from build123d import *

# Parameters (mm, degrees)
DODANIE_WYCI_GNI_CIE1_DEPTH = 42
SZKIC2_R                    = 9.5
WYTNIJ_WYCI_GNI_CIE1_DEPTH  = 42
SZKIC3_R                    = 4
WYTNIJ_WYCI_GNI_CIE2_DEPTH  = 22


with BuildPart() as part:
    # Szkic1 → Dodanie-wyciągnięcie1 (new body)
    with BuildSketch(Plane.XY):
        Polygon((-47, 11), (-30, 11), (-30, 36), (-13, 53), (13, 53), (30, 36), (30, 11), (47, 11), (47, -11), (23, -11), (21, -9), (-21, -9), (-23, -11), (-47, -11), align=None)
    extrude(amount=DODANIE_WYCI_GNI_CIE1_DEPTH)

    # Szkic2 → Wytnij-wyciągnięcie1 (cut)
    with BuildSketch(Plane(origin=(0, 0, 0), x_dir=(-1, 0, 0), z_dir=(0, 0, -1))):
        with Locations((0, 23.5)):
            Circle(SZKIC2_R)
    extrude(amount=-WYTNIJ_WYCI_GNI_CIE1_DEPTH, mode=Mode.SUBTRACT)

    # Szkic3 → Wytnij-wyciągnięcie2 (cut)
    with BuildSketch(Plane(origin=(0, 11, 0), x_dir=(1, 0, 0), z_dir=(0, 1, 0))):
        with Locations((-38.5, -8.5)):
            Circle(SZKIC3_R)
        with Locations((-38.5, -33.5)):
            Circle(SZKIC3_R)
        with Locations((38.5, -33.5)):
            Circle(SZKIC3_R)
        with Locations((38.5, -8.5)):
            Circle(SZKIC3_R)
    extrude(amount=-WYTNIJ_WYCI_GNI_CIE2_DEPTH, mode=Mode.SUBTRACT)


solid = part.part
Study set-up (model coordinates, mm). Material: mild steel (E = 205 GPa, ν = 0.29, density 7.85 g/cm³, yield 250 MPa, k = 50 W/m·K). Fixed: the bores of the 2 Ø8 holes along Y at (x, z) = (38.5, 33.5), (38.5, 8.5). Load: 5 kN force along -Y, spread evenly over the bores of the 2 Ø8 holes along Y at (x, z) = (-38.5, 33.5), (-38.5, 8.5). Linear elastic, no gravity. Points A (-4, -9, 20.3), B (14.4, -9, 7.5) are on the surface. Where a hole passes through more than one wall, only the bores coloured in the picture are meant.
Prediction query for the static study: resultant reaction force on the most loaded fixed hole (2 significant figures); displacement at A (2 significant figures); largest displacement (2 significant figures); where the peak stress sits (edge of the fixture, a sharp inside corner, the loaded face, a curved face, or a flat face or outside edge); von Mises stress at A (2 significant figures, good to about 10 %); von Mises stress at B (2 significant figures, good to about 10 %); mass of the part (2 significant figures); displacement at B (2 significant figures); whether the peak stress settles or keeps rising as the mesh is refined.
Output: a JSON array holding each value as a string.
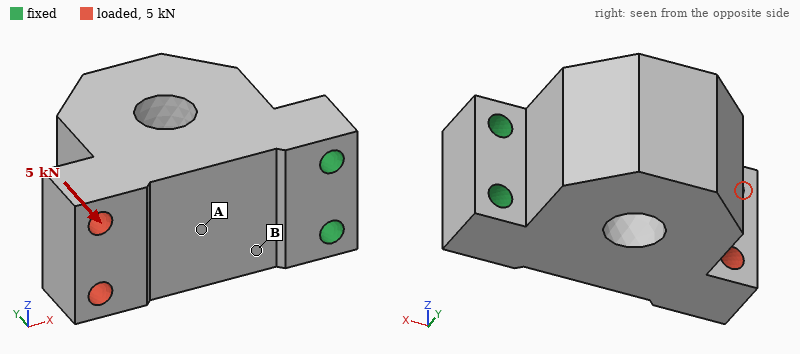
["2.5 kN", "34 µm", "83 µm", "edge of the fixture", "20 MPa", "52 MPa", "1.3 kg", "16 µm", "keeps rising"]
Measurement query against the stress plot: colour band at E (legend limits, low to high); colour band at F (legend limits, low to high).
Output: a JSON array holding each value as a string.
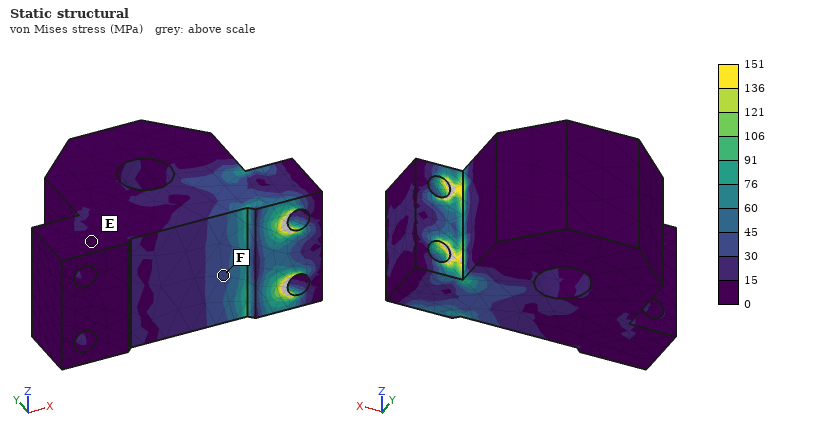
["0 to 15 MPa", "30 to 45 MPa"]
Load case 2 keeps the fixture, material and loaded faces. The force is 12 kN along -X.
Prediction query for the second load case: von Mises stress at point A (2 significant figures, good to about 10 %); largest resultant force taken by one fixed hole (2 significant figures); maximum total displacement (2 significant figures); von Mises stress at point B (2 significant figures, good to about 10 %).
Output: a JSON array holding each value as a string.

["18 MPa", "6.1 kN", "10 µm", "20 MPa"]
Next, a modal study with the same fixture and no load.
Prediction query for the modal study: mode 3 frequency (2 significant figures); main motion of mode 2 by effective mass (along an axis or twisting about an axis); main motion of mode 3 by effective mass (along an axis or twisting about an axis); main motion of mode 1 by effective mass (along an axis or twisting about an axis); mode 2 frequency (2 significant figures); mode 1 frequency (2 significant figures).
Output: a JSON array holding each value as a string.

["4800 Hz", "along Z", "twisting about X", "along Y", "3300 Hz", "1900 Hz"]
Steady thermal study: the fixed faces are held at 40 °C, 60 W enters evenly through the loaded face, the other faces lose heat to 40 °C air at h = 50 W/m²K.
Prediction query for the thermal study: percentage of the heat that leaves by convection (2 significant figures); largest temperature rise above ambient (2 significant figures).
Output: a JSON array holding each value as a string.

["44 %", "61 K"]
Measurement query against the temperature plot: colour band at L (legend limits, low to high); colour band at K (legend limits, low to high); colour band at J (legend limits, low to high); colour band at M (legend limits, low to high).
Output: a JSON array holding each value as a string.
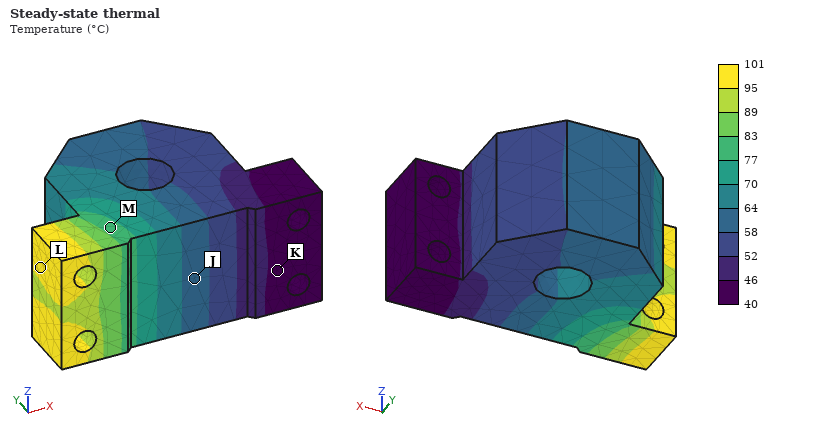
["95 to 101 °C", "40 to 46 °C", "58 to 64 °C", "77 to 83 °C"]
